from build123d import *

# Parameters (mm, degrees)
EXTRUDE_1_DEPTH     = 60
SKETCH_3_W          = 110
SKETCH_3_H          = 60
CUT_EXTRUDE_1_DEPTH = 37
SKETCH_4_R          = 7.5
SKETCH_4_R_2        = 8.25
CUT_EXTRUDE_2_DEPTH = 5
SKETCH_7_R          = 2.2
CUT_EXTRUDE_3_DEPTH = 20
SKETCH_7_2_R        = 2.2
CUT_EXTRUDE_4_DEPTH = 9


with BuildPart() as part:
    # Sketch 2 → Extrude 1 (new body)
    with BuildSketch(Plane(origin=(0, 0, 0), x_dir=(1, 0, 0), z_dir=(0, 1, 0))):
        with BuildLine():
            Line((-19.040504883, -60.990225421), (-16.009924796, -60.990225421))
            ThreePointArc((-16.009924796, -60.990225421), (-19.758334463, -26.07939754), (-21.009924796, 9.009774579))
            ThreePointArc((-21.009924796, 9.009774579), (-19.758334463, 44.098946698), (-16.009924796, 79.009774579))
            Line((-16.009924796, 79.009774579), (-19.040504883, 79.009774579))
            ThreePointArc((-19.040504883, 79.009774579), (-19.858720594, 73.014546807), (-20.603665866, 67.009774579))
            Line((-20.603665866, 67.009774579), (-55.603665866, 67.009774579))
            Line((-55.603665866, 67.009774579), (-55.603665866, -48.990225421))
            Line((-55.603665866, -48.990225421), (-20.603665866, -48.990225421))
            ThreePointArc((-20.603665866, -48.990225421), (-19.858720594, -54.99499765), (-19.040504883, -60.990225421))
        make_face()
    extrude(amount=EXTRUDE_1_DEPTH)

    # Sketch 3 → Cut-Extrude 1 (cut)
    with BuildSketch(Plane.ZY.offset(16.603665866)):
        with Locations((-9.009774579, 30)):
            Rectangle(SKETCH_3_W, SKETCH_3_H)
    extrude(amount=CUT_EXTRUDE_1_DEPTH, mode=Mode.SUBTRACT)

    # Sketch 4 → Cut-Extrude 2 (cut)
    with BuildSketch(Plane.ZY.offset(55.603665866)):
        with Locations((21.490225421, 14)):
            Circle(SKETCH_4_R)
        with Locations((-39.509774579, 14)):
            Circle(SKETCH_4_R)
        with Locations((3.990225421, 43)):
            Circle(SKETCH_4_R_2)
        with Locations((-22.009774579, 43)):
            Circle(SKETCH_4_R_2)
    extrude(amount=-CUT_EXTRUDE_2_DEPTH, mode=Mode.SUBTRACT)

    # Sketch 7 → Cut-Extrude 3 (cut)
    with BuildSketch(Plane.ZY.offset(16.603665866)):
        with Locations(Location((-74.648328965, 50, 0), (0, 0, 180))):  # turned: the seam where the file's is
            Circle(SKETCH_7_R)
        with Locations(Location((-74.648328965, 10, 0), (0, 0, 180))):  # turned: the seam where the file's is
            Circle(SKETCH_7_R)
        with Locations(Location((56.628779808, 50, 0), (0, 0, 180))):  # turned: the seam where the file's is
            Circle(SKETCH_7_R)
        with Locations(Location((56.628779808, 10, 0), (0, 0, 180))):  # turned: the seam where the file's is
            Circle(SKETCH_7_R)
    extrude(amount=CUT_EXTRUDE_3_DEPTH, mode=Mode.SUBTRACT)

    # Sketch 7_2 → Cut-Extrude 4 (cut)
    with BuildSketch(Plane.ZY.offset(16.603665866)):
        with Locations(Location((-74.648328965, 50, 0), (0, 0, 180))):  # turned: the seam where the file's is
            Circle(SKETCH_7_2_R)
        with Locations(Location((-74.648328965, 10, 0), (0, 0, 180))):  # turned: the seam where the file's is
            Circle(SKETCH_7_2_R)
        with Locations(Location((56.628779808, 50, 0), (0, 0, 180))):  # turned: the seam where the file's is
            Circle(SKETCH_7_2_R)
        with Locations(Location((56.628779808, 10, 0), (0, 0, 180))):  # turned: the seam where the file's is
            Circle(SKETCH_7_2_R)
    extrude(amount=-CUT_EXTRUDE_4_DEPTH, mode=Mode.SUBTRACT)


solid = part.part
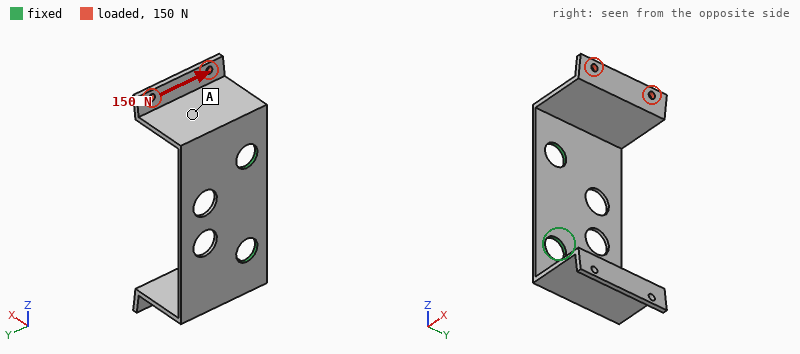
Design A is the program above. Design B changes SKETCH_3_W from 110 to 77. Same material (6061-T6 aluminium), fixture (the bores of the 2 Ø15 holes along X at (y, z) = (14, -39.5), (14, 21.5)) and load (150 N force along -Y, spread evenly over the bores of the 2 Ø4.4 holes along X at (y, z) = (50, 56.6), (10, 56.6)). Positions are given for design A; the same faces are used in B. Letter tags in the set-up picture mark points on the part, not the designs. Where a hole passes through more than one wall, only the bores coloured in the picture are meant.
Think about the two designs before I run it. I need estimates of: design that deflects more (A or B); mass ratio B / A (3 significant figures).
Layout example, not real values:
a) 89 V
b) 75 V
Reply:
a) A
b) 3.34
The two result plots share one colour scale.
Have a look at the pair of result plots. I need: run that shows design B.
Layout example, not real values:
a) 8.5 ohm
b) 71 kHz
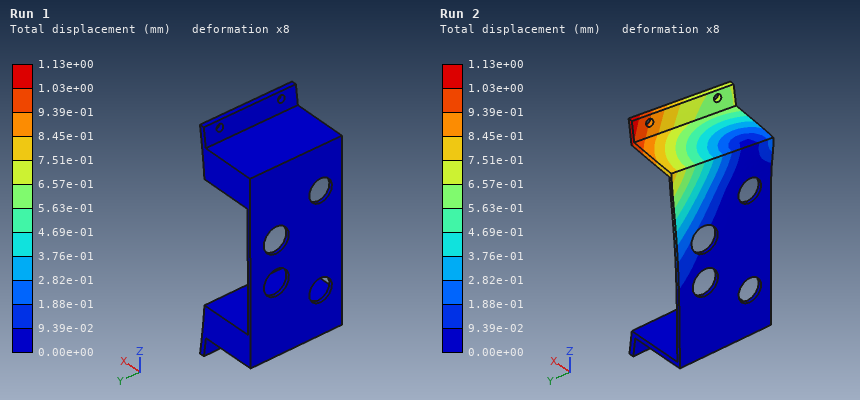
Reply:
a) Run 1
